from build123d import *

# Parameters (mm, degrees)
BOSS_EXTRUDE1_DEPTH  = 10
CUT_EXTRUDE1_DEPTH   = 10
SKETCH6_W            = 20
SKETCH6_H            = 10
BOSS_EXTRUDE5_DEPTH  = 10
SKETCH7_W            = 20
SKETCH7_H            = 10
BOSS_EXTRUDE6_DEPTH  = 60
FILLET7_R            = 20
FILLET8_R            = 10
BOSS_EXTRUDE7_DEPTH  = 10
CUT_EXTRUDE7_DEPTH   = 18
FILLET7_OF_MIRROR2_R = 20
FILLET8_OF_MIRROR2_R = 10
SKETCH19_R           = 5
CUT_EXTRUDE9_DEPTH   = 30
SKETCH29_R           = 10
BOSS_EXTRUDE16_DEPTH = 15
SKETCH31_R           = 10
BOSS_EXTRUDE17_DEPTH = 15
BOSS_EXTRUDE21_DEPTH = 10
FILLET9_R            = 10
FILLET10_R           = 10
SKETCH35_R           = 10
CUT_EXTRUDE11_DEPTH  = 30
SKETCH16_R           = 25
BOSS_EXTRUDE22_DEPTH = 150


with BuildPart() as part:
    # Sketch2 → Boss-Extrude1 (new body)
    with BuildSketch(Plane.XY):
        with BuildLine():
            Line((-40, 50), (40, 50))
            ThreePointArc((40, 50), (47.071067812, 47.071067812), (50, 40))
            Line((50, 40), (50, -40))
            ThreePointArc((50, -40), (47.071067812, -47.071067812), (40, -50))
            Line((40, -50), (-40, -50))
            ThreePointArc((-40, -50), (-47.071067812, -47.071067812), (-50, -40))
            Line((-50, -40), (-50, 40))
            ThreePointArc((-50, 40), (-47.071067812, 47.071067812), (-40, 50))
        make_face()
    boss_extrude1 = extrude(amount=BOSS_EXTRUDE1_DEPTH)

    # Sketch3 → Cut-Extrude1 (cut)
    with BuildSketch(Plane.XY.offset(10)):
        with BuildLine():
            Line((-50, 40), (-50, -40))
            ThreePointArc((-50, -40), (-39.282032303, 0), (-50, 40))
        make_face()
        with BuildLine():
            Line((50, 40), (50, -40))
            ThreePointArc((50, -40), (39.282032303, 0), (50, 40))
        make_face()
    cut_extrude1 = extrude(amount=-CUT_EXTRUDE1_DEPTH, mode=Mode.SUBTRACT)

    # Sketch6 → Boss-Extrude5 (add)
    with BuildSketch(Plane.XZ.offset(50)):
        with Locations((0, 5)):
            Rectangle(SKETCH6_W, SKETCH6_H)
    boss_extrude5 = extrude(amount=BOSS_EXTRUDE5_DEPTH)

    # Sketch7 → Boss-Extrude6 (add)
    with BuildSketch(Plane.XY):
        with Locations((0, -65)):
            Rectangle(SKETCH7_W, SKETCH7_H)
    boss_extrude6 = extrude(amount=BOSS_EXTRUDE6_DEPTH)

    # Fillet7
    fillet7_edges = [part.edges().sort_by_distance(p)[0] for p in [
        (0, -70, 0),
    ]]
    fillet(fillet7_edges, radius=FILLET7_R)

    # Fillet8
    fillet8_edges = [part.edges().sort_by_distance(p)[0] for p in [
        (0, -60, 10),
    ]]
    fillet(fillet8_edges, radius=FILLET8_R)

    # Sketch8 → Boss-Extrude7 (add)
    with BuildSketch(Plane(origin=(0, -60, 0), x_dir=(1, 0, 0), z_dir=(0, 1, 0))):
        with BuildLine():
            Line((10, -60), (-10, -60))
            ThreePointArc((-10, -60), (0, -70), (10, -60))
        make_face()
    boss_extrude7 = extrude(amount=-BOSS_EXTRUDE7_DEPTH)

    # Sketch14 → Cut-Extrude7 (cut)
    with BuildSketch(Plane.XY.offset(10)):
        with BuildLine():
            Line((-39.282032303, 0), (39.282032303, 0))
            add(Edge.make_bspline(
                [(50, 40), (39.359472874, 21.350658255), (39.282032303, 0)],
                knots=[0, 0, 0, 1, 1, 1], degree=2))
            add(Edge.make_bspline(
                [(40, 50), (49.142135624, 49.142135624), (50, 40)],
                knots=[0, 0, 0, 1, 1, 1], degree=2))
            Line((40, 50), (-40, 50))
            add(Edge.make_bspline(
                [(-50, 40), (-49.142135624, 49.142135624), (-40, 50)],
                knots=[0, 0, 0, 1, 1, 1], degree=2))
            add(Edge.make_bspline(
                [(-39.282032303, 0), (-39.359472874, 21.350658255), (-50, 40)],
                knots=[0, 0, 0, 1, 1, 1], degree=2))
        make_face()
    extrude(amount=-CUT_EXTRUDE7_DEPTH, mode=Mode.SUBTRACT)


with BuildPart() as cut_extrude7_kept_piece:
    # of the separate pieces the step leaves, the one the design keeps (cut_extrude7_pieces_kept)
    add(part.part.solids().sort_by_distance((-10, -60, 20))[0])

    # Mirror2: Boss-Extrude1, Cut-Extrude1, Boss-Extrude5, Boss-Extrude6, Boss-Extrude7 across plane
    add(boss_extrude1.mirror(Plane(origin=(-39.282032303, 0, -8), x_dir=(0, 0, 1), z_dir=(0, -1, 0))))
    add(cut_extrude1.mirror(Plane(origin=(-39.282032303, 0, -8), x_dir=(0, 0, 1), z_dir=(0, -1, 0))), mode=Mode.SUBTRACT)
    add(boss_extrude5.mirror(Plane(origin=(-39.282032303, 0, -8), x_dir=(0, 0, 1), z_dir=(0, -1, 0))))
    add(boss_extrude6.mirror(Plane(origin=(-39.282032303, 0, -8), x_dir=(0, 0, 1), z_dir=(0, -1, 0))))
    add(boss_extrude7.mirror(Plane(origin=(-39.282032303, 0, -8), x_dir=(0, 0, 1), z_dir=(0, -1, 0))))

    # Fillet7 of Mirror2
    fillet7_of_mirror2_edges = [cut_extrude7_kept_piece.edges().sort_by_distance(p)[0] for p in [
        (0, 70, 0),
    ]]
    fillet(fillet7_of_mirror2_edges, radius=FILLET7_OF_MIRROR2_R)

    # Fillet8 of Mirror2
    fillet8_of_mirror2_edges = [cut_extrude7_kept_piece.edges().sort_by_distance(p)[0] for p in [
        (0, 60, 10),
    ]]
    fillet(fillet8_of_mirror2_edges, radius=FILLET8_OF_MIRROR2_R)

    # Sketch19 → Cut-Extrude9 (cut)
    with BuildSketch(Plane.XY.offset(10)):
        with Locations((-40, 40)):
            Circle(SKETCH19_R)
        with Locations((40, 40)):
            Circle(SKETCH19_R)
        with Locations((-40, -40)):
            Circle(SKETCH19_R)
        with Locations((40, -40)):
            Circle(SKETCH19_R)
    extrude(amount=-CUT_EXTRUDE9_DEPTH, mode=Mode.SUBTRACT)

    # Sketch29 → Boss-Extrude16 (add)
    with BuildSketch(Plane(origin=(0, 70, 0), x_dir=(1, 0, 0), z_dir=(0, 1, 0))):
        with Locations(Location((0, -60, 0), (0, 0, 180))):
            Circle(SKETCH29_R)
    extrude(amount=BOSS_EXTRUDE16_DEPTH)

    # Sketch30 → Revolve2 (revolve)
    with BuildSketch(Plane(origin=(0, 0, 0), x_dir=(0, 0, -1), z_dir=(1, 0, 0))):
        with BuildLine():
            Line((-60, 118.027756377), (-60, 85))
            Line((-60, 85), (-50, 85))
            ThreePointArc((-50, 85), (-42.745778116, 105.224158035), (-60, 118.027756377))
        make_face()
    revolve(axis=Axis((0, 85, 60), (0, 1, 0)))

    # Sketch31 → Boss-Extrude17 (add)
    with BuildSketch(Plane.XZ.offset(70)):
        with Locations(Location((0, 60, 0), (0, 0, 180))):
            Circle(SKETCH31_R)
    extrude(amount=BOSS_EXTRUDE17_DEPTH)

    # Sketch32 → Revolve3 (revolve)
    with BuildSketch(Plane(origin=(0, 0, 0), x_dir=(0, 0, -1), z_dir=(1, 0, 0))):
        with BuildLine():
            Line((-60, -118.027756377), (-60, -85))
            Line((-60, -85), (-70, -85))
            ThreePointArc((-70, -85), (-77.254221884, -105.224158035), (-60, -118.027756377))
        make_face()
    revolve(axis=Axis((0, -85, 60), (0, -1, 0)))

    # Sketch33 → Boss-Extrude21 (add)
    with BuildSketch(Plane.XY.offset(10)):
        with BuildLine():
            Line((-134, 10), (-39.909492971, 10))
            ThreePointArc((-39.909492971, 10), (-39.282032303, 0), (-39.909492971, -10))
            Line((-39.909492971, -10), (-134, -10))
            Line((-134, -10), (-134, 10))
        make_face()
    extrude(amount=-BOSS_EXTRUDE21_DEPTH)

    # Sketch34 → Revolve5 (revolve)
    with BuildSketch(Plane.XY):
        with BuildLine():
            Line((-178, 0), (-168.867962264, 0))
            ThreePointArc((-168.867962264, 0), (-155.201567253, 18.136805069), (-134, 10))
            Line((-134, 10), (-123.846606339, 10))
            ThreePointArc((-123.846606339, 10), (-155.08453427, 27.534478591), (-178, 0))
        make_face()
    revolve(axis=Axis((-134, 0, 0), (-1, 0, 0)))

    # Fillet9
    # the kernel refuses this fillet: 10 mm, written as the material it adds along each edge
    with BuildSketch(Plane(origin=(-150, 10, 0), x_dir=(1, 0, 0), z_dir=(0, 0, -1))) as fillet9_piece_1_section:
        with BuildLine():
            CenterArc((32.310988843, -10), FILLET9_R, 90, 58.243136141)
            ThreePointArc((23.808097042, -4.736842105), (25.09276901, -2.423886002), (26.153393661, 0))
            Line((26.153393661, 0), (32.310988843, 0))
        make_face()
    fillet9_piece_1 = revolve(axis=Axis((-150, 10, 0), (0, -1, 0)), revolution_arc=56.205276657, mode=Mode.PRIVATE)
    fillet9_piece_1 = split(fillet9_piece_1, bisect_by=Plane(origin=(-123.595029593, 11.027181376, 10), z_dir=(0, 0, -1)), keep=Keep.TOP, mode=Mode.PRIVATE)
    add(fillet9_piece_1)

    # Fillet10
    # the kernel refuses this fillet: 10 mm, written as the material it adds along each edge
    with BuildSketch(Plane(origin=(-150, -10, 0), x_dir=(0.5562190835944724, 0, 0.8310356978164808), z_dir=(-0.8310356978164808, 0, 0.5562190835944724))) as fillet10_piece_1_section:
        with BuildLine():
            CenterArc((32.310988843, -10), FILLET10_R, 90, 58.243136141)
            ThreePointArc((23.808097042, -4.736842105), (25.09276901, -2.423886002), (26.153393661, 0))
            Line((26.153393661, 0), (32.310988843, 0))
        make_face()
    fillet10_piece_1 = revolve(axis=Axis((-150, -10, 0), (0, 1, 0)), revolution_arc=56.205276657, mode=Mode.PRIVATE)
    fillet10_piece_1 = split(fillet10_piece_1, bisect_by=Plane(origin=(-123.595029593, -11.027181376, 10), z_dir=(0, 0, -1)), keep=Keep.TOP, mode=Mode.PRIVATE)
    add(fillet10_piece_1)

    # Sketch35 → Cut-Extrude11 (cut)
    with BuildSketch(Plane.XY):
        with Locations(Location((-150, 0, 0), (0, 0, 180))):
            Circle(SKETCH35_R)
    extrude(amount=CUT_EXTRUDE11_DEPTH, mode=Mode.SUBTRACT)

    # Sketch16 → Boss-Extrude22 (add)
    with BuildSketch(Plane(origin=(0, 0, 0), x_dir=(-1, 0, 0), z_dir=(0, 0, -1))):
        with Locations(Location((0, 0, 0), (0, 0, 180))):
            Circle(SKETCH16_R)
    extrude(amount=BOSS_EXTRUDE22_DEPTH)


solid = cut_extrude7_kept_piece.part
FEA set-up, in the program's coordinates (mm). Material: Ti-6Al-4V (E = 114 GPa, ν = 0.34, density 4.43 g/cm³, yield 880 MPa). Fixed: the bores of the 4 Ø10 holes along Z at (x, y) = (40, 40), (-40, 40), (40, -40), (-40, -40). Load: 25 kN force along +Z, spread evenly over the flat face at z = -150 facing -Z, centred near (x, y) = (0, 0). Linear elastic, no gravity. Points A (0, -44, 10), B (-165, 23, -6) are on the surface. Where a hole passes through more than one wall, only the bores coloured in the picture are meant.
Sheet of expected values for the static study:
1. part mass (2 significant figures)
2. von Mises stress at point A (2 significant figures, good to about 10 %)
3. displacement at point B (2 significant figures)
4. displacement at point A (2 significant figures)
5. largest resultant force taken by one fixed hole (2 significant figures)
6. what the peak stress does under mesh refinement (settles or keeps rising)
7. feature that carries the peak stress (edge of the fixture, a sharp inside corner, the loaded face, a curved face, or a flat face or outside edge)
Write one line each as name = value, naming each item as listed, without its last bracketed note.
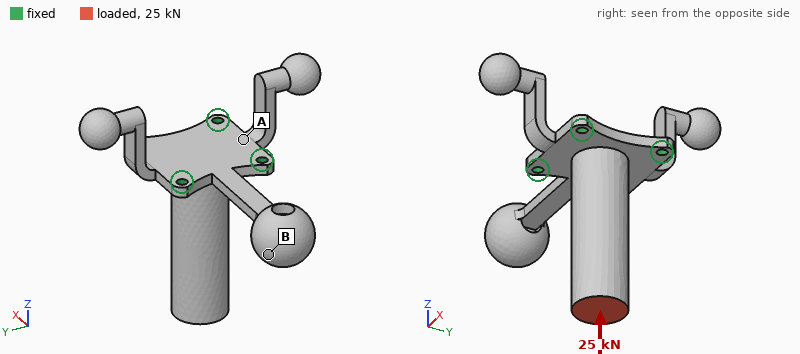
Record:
part mass = 2.4 kg
von Mises stress at point A = 52 MPa
displacement at point B = 0.068 mm
displacement at point A = 0.040 mm
largest resultant force taken by one fixed hole = 6.5 kN
what the peak stress does under mesh refinement = keeps rising
feature that carries the peak stress = edge of the fixture
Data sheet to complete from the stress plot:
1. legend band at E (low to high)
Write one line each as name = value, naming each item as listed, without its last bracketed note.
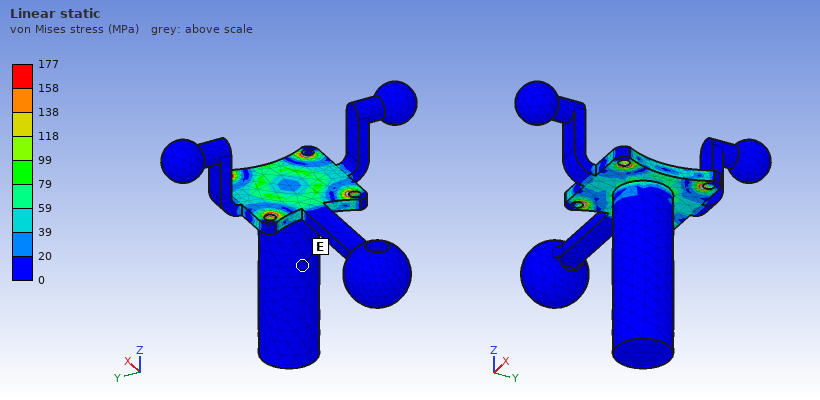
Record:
legend band at E = 0 to 20 MPa
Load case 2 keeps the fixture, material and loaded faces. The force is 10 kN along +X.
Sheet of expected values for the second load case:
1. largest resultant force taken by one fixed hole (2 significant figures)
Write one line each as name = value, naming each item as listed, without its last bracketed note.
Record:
largest resultant force taken by one fixed hole = 12 kN
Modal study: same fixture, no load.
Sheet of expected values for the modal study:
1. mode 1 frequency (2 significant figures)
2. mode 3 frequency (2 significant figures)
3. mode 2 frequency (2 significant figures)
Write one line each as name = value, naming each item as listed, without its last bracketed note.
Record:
mode 1 frequency = 170 Hz
mode 3 frequency = 380 Hz
mode 2 frequency = 340 Hz
